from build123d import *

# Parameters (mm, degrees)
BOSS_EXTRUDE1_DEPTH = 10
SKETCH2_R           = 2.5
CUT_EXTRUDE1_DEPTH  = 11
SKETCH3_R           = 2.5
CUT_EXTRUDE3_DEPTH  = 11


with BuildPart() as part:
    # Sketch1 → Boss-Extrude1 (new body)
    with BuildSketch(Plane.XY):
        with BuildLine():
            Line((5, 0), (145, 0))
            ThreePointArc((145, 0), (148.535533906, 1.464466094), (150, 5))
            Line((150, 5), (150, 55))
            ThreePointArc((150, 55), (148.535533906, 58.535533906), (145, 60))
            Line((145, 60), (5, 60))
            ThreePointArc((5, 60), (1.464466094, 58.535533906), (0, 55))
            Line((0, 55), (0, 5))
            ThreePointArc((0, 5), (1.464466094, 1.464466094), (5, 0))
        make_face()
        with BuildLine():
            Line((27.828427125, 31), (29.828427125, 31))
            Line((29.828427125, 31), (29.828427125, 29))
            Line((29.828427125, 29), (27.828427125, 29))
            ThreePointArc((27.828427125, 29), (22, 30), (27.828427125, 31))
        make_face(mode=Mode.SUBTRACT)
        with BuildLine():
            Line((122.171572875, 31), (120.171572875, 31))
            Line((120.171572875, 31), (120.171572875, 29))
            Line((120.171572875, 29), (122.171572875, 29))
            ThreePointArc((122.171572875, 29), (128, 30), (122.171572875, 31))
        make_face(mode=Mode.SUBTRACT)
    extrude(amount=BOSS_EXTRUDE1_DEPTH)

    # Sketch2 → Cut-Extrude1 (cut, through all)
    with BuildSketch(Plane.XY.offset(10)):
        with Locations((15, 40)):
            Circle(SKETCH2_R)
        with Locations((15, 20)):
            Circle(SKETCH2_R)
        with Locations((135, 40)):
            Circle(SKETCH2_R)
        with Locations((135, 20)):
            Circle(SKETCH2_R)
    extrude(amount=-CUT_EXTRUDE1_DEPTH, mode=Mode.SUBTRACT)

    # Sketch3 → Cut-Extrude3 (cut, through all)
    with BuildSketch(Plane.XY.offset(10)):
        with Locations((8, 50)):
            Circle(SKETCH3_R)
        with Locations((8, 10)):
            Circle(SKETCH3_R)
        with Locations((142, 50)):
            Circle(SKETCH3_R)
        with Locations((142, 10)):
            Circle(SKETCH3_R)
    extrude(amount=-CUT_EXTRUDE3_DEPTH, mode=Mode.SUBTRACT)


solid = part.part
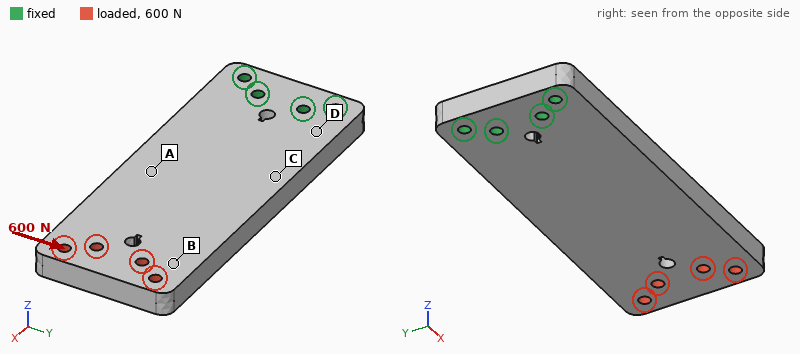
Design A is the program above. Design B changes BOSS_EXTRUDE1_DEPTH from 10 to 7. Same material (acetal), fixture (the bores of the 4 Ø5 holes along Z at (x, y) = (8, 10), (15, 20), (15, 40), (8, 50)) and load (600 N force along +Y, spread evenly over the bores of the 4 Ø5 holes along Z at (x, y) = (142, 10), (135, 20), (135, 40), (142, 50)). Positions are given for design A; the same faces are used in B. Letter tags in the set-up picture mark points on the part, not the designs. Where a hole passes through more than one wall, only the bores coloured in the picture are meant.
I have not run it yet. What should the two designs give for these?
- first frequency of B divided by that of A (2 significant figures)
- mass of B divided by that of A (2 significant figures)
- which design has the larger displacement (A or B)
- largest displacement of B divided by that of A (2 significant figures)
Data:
0.71
0.70
B
1.4
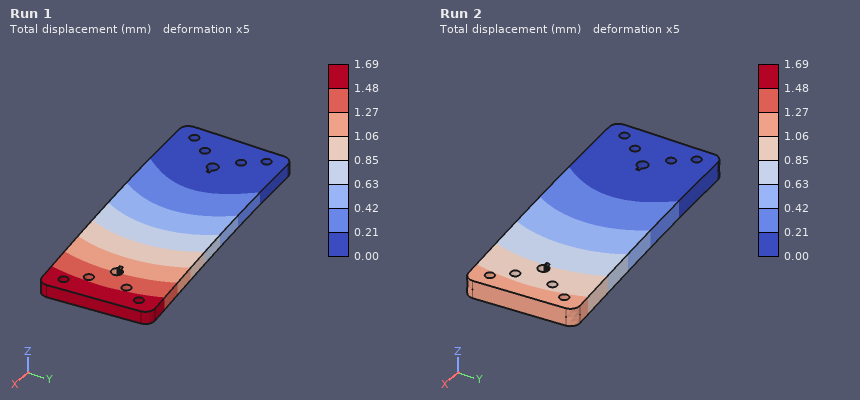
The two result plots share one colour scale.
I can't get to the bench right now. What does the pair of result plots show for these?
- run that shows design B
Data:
Run 1
